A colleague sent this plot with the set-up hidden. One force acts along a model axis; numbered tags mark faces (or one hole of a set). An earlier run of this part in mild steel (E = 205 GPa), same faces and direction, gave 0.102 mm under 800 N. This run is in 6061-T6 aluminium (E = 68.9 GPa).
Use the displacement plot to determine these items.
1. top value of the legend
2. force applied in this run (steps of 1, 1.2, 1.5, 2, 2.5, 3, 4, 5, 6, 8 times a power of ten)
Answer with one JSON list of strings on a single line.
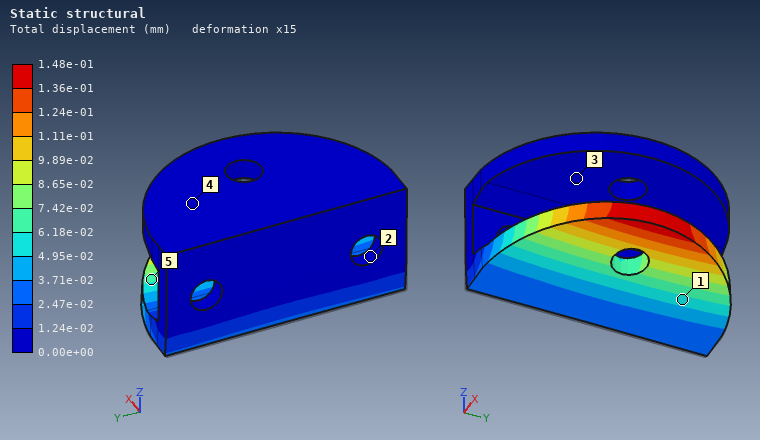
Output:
["1.48e-01 mm", "400 N"]
